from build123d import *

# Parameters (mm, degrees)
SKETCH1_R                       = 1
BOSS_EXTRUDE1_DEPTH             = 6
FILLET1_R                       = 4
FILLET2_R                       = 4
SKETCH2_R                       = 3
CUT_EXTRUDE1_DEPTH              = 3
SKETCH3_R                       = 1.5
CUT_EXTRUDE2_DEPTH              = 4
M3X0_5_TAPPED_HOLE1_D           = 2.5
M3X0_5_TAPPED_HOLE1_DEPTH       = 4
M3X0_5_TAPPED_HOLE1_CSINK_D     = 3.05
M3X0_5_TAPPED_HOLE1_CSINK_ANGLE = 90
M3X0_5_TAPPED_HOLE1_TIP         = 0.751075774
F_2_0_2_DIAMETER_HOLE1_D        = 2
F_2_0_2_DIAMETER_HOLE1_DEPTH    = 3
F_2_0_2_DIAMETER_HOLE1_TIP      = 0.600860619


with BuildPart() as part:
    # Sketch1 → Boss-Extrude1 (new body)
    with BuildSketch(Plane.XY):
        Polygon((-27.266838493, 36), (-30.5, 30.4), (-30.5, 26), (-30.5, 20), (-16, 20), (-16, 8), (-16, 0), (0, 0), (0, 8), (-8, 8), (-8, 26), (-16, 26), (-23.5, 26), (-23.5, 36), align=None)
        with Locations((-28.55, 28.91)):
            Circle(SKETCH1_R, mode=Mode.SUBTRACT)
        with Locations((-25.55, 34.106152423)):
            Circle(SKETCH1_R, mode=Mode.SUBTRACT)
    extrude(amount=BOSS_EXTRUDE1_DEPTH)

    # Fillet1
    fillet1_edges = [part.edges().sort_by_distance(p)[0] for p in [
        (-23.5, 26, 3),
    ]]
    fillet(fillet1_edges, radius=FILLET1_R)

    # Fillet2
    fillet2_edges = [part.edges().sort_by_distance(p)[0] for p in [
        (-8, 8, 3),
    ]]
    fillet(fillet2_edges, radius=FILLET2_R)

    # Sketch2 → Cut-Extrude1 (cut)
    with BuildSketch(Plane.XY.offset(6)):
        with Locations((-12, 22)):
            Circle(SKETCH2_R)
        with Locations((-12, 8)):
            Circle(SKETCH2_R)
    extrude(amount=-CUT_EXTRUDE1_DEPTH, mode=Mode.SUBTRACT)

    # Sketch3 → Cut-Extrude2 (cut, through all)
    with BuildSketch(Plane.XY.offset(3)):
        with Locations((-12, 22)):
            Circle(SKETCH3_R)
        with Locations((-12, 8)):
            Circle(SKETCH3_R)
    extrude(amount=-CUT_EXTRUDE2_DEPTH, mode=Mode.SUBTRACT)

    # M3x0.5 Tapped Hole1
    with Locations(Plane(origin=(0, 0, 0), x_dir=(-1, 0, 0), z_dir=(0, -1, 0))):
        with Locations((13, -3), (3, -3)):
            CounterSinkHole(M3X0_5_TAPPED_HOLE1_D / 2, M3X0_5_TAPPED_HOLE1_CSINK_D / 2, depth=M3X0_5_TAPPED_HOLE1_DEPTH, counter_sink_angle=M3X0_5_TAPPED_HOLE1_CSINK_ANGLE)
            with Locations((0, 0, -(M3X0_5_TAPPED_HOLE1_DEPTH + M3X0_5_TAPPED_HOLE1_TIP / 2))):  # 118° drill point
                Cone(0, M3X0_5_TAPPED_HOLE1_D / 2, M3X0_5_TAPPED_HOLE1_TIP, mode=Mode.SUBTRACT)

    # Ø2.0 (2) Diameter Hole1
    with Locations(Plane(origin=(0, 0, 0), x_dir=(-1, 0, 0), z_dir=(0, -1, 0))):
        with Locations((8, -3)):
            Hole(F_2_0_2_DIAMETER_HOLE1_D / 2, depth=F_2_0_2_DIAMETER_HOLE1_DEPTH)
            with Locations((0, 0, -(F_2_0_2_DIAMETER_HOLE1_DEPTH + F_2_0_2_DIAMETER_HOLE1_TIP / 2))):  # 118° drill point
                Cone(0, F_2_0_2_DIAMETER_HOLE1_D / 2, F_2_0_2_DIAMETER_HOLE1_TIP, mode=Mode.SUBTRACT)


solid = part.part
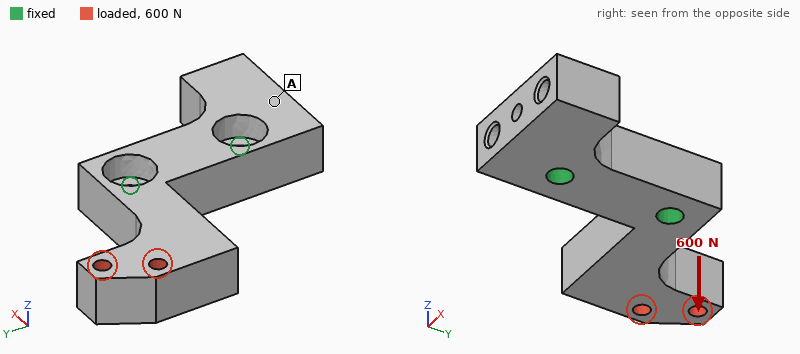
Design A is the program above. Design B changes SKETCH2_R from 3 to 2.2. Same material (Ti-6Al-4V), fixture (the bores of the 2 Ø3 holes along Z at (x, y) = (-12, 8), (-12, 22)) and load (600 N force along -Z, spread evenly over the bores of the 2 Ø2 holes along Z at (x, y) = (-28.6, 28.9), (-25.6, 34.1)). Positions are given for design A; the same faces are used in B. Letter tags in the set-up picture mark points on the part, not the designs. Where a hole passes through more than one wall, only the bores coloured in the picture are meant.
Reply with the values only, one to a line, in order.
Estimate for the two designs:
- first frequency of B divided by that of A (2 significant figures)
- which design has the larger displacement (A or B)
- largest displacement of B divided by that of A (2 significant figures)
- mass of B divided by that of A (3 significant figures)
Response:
1.1
A
0.89
1.03
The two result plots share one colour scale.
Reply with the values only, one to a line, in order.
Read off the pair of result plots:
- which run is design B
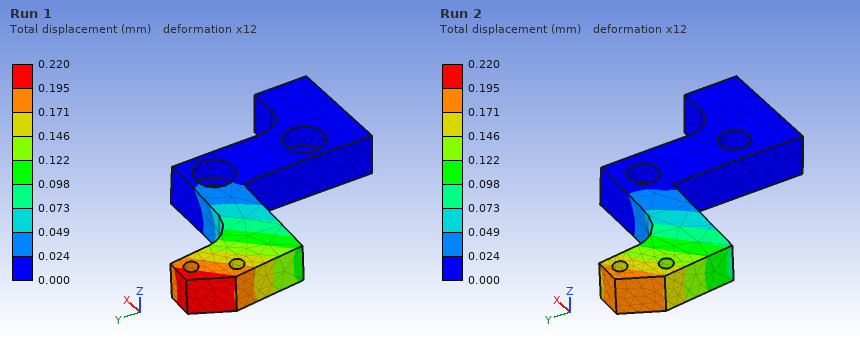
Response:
Run 2
